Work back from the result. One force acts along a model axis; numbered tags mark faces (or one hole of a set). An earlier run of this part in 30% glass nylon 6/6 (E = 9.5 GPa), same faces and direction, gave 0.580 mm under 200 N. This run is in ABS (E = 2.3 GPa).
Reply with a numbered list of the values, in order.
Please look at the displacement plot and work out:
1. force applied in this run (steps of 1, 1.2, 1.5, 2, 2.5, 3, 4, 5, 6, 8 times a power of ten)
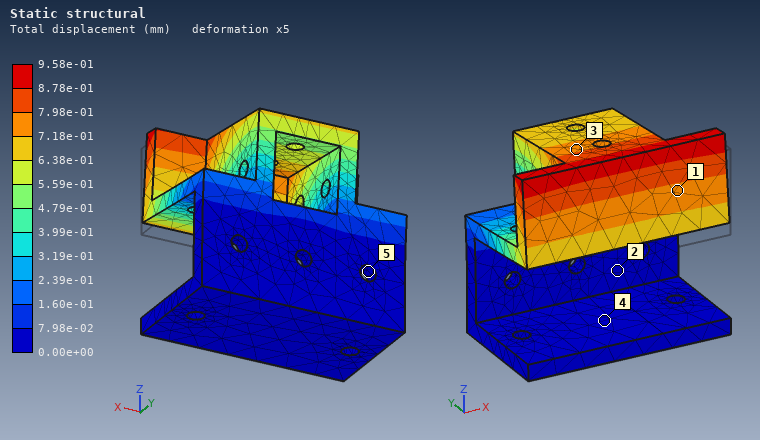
1. 80 N
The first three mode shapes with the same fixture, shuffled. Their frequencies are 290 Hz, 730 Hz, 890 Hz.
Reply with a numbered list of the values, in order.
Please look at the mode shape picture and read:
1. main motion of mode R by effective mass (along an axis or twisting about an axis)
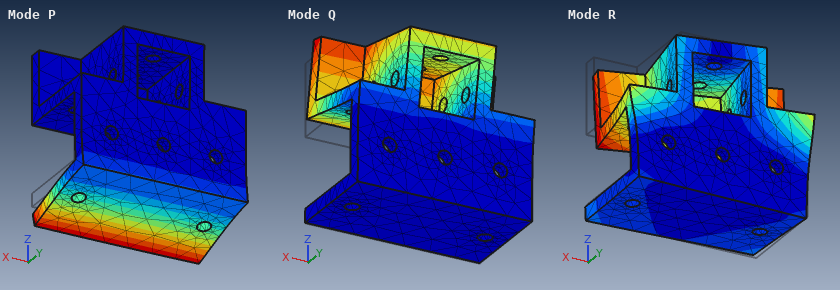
1. along X
